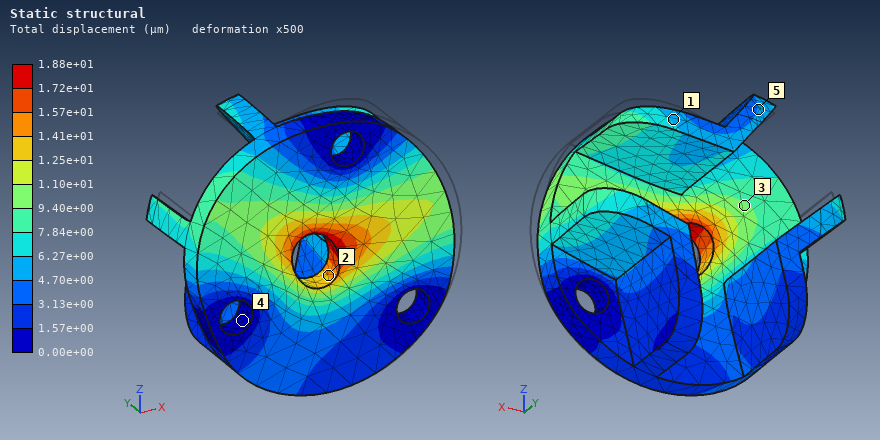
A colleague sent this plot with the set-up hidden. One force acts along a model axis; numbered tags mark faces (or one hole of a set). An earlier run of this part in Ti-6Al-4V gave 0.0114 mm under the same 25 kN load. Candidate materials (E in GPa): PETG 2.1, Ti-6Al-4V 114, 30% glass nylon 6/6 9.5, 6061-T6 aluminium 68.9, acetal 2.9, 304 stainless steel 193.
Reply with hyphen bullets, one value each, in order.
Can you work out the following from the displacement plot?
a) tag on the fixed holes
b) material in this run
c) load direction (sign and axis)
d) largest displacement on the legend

- 4
- 6061-T6 aluminium
- -X
- 1.88e+01 µm
